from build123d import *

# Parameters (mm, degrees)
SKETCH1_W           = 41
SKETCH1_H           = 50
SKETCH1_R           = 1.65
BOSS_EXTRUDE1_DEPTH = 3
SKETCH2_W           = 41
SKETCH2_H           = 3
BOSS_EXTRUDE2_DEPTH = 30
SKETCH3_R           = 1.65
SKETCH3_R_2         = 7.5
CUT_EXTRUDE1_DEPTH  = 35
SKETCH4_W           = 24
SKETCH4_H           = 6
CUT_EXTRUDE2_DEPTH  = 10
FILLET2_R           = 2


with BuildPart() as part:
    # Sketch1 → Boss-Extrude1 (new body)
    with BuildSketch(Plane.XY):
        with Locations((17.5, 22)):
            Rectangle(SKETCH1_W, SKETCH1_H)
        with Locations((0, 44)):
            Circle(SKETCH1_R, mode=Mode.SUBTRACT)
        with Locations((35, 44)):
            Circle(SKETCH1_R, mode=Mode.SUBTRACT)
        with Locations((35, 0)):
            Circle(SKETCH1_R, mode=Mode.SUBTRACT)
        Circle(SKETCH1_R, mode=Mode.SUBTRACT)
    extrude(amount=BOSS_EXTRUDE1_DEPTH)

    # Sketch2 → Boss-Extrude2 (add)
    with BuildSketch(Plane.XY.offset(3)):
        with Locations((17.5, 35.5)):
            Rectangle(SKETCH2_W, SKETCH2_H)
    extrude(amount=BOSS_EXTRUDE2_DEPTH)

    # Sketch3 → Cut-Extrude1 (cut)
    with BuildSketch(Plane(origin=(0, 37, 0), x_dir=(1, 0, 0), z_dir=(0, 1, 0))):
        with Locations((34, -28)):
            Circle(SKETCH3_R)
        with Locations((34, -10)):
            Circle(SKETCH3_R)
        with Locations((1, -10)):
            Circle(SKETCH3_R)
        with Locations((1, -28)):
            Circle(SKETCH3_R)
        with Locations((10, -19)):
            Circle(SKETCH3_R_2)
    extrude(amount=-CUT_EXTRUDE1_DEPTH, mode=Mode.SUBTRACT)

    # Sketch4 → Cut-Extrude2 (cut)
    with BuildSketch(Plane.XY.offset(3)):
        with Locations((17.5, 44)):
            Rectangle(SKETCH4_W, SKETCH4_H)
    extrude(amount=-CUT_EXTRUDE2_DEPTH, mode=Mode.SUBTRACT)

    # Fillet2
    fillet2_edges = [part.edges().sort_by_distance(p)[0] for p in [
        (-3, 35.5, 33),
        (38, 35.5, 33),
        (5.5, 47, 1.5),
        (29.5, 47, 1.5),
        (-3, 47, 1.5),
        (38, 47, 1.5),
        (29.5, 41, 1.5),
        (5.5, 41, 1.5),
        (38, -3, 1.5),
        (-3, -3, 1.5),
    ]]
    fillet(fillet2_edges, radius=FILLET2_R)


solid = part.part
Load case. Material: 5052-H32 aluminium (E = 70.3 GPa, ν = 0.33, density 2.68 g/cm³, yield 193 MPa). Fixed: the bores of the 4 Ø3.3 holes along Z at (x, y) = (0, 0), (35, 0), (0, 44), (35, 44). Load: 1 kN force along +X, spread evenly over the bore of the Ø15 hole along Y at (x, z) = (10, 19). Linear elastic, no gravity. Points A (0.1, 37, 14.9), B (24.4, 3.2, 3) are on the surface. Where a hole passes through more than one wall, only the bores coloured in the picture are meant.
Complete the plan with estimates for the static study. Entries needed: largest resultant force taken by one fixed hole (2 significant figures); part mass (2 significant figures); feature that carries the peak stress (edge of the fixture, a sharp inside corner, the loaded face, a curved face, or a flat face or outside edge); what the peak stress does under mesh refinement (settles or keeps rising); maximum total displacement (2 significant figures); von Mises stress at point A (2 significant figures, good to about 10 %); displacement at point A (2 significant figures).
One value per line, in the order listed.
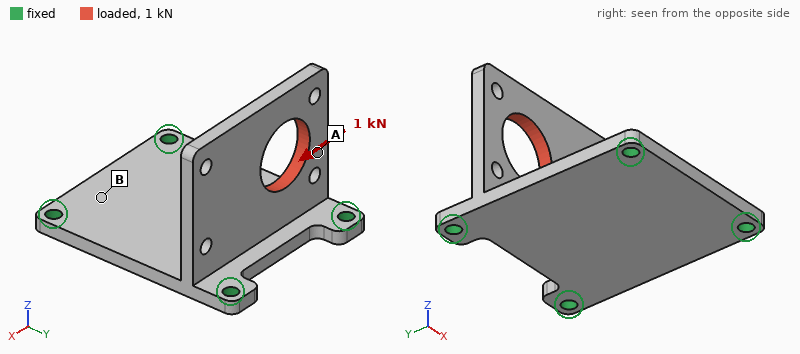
620 N
23 g
edge of the fixture
keeps rising
83 µm
31 MPa
48 µm
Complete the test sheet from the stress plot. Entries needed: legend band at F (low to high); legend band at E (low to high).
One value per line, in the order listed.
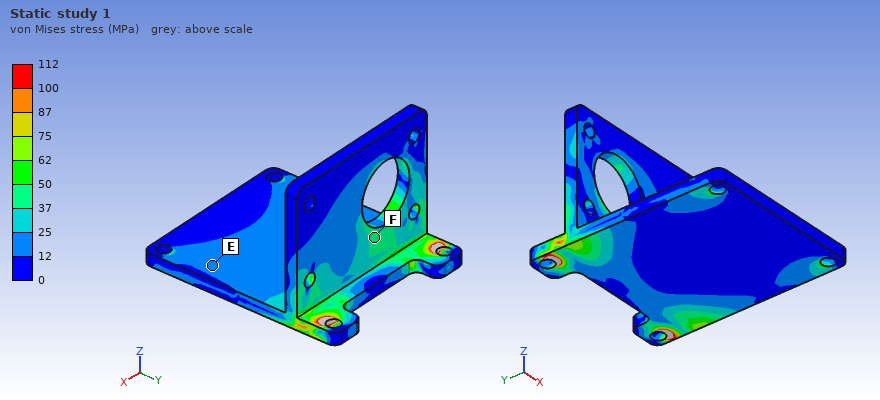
37 to 50 MPa
12 to 25 MPa
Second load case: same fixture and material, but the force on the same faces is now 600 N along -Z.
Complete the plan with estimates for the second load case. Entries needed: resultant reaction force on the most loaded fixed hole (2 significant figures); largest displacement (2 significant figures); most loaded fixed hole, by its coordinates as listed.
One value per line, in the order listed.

390 N
63 µm
(0, 44)
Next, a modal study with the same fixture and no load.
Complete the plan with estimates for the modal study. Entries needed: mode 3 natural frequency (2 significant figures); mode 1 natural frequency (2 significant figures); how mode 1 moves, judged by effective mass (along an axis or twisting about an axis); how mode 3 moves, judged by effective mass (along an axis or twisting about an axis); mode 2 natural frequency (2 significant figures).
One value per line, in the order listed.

6400 Hz
2100 Hz
along Y
along Z
4400 Hz
